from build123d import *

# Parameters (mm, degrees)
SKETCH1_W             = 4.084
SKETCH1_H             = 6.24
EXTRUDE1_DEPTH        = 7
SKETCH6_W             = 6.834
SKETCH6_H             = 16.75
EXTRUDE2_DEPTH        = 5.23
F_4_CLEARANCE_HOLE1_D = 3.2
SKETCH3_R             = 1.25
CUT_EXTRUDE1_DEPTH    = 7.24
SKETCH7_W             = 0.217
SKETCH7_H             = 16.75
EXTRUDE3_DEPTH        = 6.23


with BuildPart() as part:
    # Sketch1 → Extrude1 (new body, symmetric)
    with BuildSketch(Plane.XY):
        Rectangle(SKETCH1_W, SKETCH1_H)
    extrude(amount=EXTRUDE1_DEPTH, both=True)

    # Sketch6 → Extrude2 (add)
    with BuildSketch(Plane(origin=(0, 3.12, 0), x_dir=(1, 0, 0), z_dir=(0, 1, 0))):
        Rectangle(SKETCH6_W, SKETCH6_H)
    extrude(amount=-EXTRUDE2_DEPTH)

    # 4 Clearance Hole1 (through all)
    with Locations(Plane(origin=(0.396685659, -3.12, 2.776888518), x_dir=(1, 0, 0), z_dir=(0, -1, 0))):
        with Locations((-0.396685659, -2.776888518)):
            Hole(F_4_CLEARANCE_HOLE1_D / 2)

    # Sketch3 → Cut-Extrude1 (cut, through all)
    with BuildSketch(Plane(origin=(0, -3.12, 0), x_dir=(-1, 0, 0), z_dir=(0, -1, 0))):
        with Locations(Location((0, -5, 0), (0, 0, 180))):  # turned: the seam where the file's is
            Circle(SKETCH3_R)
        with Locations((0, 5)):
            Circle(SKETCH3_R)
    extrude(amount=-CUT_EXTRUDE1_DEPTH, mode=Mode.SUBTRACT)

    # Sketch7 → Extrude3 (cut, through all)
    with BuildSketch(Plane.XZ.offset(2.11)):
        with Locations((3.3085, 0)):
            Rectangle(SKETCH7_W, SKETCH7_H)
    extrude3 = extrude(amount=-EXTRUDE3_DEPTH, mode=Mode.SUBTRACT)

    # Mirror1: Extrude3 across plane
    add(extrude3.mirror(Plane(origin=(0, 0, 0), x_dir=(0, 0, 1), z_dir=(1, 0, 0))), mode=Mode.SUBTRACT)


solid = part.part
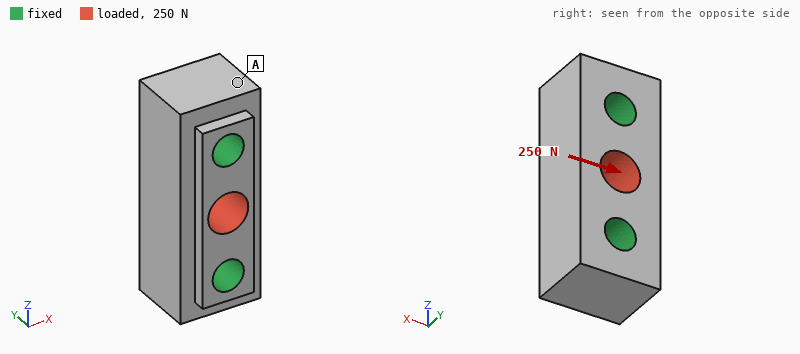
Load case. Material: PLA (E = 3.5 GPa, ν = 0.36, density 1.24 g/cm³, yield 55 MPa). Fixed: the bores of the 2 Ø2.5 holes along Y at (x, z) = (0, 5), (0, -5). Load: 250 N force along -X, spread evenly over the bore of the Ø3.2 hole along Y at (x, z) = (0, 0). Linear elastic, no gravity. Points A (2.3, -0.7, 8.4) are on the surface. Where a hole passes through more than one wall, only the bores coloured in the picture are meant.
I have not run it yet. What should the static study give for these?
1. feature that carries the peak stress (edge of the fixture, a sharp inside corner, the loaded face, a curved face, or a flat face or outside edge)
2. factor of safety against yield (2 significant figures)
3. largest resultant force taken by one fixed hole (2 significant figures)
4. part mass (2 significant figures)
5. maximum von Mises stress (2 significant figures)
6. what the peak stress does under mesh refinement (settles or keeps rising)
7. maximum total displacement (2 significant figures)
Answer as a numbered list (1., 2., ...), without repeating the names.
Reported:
1. a flat face or outside edge
2. 2.2
3. 130 N
4. 0.63 g
5. 25 MPa
6. settles
7. 25 µm
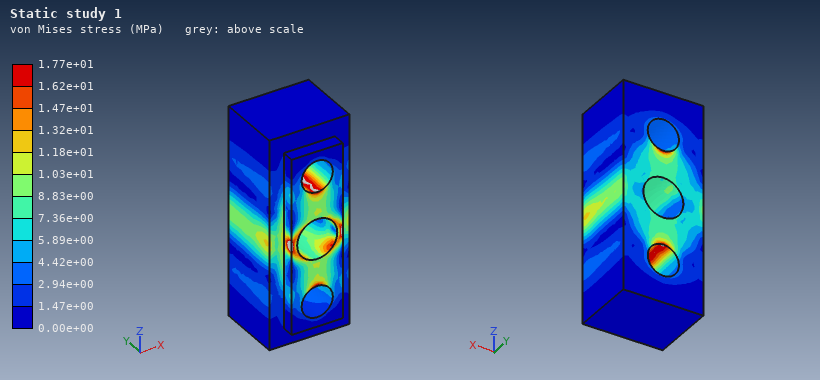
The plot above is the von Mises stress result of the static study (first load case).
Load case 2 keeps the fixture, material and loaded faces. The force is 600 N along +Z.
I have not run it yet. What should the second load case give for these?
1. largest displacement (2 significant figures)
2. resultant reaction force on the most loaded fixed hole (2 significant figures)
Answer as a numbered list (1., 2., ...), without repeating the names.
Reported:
1. 14 µm
2. 300 N
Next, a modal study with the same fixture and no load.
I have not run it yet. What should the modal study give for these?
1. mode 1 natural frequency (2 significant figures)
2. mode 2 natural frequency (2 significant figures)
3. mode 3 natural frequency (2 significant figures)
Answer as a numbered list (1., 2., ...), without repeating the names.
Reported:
1. 52 kHz
2. 55 kHz
3. 56 kHz
